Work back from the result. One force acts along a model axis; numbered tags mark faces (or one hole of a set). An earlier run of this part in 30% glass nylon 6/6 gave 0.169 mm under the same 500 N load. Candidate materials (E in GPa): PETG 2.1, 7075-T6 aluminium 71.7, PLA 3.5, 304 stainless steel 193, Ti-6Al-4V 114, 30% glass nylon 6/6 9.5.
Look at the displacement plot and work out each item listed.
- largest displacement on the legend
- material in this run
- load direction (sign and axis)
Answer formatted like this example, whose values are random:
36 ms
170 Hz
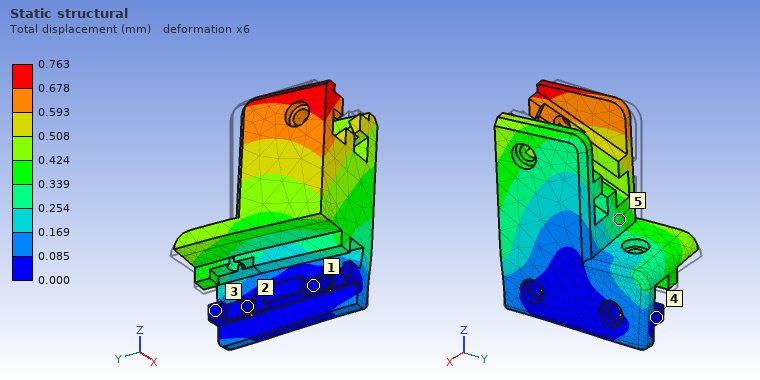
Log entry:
0.763 mm
PETG
-Y
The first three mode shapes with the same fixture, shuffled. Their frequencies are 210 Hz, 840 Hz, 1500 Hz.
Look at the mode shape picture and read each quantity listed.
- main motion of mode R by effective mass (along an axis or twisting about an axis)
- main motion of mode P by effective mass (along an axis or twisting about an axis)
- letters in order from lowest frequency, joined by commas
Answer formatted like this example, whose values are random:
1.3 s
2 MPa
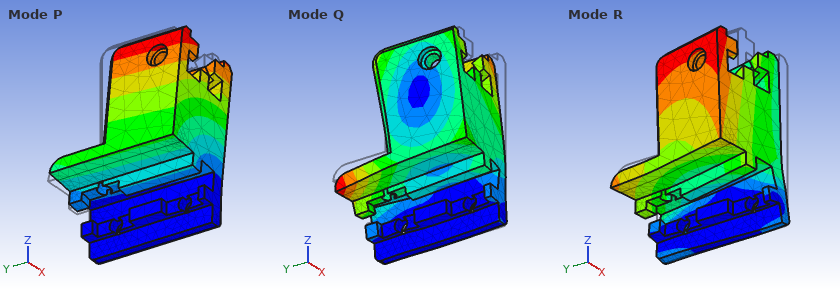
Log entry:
along Y
along X
P, R, Q
